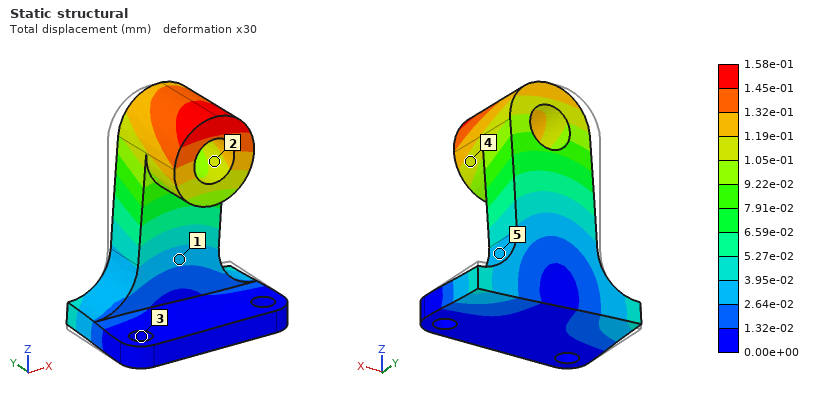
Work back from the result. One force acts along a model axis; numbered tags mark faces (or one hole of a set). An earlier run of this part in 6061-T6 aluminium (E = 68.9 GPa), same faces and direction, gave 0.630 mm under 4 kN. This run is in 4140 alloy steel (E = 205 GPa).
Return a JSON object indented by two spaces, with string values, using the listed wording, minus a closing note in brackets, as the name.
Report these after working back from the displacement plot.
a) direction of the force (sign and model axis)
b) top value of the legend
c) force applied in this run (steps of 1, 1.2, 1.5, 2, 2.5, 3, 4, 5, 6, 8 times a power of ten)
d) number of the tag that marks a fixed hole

{
  "direction of the force": "+X",
  "top value of the legend": "1.58e-01 mm",
  "force applied in this run": "3 kN",
  "number of the tag that marks a fixed hole": "3"
}
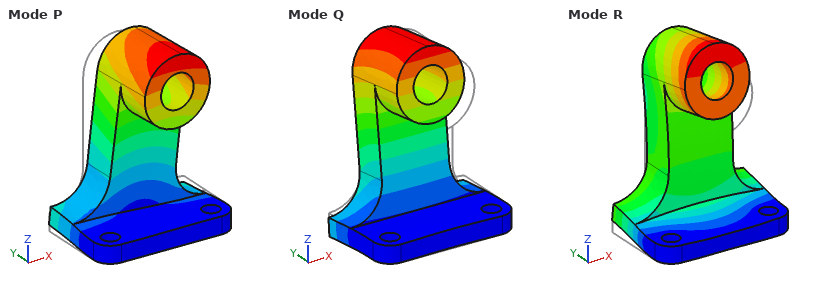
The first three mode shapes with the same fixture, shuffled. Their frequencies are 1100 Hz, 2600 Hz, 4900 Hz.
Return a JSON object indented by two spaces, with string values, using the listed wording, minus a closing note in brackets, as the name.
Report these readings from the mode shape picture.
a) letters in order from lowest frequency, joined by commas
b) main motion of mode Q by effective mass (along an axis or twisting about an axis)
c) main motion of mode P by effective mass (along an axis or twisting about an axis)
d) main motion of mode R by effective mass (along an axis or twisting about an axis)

{
  "letters in order from lowest frequency, joined by commas": "Q, P, R",
  "main motion of mode Q by effective mass": "along Y",
  "main motion of mode P by effective mass": "along X",
  "main motion of mode R by effective mass": "along Z"
}
